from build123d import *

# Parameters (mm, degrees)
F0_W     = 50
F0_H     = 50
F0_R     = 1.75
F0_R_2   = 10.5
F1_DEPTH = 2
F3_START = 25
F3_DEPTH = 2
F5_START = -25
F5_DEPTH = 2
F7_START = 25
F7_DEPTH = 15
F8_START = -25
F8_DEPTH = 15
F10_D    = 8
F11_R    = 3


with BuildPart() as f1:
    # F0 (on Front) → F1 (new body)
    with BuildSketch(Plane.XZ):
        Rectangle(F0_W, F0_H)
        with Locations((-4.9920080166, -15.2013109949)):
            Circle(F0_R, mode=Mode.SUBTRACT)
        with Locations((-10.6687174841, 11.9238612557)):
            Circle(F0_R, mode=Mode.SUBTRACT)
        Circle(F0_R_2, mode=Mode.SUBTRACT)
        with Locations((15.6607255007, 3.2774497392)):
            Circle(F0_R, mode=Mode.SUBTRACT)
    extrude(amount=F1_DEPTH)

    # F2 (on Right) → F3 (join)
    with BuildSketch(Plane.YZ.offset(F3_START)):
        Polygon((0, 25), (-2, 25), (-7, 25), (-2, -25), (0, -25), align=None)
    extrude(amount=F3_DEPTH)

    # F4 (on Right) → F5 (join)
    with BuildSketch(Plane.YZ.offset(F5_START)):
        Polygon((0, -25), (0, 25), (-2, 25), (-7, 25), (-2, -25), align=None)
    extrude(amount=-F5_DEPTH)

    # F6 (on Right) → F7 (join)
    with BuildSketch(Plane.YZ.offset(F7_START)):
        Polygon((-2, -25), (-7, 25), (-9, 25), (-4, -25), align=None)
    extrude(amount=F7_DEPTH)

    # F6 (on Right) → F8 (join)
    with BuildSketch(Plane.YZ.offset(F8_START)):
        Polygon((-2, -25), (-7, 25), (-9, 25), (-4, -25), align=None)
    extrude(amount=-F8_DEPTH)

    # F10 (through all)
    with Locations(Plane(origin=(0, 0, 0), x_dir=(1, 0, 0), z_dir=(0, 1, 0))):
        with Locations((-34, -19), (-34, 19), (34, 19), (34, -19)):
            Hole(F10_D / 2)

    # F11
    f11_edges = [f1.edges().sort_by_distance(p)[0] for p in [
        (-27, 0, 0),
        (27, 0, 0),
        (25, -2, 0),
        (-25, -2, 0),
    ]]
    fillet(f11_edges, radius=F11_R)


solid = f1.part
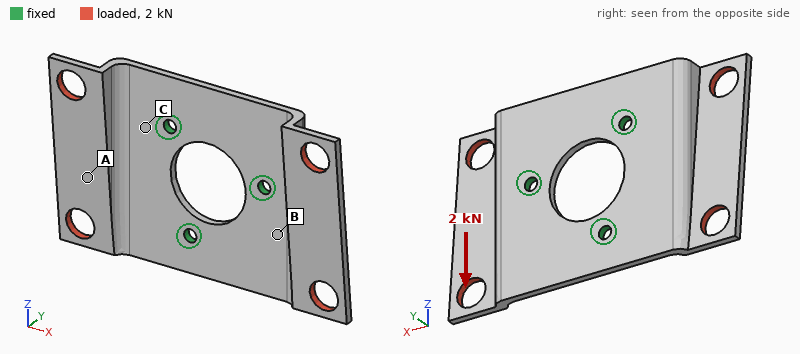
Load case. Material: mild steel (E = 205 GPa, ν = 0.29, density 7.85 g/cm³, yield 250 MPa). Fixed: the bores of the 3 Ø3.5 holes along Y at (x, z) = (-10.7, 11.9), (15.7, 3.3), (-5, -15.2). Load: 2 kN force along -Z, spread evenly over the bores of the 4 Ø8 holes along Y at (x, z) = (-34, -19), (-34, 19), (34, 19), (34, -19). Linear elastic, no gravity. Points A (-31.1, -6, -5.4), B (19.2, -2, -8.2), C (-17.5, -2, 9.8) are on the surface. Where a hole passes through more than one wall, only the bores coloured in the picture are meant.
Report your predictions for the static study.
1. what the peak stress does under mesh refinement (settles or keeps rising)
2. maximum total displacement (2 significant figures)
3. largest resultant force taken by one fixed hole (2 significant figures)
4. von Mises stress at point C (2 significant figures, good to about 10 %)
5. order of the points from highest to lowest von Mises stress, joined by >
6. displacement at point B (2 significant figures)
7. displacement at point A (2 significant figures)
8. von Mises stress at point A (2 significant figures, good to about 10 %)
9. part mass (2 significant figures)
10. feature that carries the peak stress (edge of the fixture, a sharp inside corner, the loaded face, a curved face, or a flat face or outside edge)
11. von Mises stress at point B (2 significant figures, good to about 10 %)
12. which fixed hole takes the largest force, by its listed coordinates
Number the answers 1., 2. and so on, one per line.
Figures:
1. keeps rising
2. 87 µm
3. 930 N
4. 66 MPa
5. C > B > A
6. 27 µm
7. 34 µm
8. 20 MPa
9. 61 g
10. edge of the fixture
11. 42 MPa
12. (15.7, 3.3)
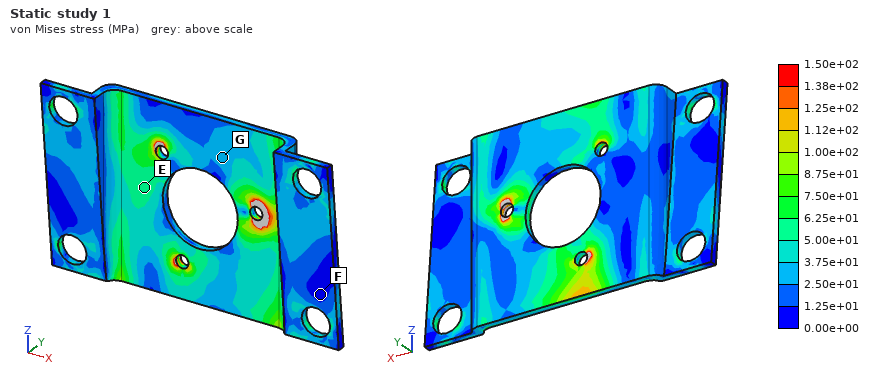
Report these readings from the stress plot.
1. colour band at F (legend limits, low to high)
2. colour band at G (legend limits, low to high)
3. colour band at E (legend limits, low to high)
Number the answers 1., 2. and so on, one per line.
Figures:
1. 0.00e+00 to 1.25e+01 MPa
2. 2.50e+01 to 3.75e+01 MPa
3. 5.00e+01 to 6.25e+01 MPa
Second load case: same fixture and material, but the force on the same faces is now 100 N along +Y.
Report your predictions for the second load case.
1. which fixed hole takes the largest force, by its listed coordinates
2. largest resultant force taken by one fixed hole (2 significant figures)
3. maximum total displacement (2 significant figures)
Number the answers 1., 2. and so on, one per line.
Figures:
1. (15.7, 3.3)
2. 72 N
3. 73 µm
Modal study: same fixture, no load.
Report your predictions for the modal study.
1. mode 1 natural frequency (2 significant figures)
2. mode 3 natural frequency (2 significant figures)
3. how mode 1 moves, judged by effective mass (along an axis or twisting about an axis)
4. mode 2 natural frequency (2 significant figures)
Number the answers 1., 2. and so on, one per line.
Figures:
1. 1600 Hz
2. 2600 Hz
3. along Y
4. 2200 Hz
